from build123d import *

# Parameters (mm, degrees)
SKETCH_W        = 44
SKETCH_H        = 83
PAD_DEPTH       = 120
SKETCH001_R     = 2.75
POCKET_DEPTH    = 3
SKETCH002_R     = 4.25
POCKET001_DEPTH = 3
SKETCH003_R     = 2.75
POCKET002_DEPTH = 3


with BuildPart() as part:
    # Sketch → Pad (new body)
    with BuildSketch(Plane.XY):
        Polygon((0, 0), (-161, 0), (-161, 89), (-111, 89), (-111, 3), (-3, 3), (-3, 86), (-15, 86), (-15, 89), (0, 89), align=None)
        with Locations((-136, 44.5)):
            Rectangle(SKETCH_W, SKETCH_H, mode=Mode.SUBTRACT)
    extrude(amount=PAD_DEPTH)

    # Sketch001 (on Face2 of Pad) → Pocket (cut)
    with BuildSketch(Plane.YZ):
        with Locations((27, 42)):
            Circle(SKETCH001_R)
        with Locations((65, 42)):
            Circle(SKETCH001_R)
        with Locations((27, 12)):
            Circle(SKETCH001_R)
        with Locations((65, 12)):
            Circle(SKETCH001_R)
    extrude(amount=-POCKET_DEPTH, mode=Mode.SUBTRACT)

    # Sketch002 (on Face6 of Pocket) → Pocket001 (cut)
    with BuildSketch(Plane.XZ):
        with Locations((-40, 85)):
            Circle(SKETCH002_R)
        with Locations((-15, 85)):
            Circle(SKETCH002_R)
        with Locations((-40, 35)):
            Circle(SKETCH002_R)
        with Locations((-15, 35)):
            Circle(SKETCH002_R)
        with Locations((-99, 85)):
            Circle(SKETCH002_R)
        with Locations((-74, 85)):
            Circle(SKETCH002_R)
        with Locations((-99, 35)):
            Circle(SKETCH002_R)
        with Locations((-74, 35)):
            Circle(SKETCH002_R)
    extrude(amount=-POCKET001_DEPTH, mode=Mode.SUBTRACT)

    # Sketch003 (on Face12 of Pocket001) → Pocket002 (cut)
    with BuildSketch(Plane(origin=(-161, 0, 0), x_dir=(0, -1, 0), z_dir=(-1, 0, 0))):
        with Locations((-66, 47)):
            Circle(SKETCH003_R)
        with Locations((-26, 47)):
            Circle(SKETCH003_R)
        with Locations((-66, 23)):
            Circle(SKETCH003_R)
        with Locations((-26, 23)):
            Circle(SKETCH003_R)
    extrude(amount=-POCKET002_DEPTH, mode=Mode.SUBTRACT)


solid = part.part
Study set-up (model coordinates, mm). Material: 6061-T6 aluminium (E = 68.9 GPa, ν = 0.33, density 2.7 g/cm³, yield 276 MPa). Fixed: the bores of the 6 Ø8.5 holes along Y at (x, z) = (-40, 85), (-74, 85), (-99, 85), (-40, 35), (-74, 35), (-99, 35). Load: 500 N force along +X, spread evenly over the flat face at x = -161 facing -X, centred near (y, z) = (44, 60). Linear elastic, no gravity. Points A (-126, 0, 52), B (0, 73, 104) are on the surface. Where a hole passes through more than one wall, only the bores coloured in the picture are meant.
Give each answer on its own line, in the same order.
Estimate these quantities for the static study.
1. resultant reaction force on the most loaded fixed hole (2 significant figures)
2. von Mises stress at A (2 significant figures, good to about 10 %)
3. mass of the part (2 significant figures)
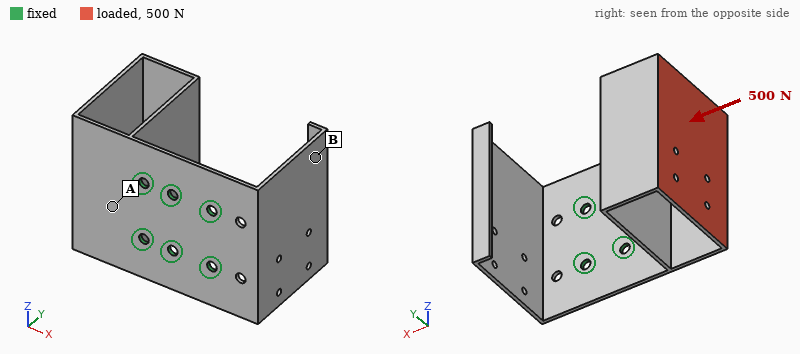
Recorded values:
210 N
40 MPa
460 g
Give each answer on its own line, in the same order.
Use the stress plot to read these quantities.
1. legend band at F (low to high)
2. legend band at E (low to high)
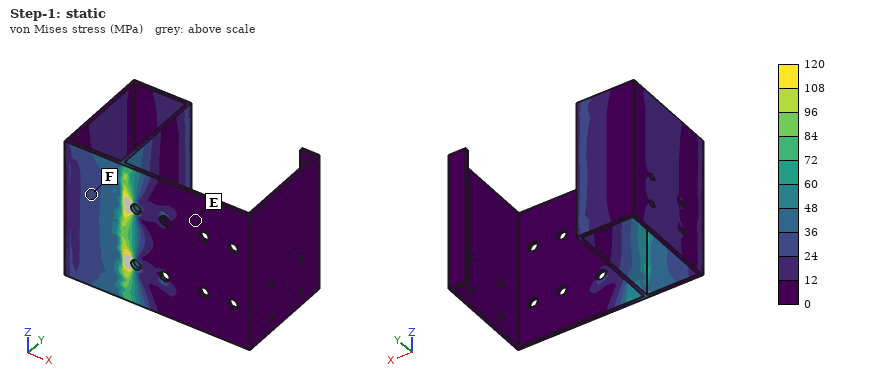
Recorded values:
24 to 36 MPa
0 to 12 MPa
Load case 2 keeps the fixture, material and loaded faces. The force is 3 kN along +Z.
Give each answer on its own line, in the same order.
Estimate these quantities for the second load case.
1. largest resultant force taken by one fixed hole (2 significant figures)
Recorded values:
3.5 kN
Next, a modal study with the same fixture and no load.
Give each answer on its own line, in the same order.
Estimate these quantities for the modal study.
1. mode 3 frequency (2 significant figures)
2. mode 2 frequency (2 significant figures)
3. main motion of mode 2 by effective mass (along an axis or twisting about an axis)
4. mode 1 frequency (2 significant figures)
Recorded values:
330 Hz
160 Hz
along X
150 Hz
